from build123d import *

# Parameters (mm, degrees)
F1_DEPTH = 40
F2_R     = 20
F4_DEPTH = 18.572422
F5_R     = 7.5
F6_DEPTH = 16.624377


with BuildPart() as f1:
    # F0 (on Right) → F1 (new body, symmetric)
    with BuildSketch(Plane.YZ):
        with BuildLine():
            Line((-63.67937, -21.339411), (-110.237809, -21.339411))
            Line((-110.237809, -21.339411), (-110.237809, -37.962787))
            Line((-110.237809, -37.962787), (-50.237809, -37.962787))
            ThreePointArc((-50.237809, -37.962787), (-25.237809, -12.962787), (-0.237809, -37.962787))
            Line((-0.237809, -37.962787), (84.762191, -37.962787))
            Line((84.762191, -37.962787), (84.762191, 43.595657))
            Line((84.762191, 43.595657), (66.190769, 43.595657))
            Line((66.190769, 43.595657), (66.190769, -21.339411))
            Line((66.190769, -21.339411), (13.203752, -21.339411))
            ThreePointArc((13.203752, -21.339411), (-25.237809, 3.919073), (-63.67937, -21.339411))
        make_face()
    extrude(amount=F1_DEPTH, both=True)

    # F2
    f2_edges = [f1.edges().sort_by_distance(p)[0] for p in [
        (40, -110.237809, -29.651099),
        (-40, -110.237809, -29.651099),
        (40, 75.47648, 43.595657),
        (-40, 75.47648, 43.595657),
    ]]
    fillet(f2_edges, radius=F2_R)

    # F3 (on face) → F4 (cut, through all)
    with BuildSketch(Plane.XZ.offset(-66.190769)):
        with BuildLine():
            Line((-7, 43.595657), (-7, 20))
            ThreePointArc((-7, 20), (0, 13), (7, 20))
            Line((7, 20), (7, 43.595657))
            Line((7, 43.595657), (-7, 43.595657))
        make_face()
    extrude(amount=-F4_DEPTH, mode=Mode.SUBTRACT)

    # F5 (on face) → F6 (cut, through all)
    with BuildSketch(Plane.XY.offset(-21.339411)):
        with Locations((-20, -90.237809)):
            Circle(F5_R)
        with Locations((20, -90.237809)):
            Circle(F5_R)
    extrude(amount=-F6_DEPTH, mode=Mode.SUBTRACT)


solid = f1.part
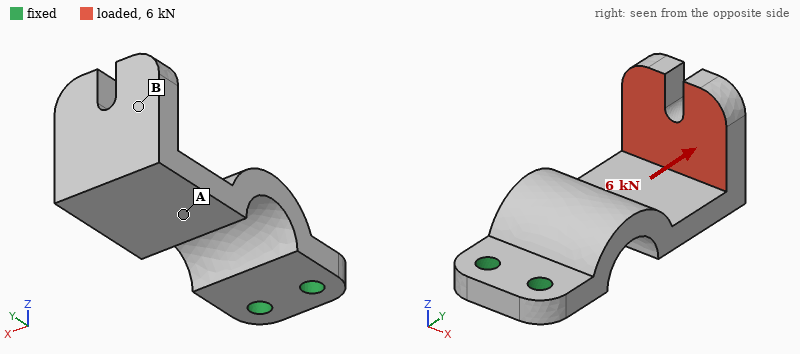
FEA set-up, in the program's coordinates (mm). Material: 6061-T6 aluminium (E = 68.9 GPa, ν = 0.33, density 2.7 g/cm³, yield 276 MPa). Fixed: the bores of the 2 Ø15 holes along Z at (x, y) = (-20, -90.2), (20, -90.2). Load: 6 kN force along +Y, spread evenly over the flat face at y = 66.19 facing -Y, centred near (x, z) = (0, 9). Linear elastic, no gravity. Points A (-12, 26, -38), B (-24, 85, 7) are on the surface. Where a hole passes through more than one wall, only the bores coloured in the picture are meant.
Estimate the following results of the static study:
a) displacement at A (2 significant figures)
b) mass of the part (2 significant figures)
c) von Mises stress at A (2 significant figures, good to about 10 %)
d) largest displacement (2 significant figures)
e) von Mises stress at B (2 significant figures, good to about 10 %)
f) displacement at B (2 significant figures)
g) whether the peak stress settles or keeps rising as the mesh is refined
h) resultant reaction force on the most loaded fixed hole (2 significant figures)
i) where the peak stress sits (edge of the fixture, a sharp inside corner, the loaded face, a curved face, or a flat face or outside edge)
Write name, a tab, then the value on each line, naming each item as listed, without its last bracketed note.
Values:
displacement at A	0.56 mm
mass of the part	1000 g
von Mises stress at A	51 MPa
largest displacement	1.7 mm
von Mises stress at B	11 MPa
displacement at B	1.4 mm
whether the peak stress settles or keeps rising as the mesh is refined	keeps rising
resultant reaction force on the most loaded fixed hole	3.1 kN
where the peak stress sits	edge of the fixture
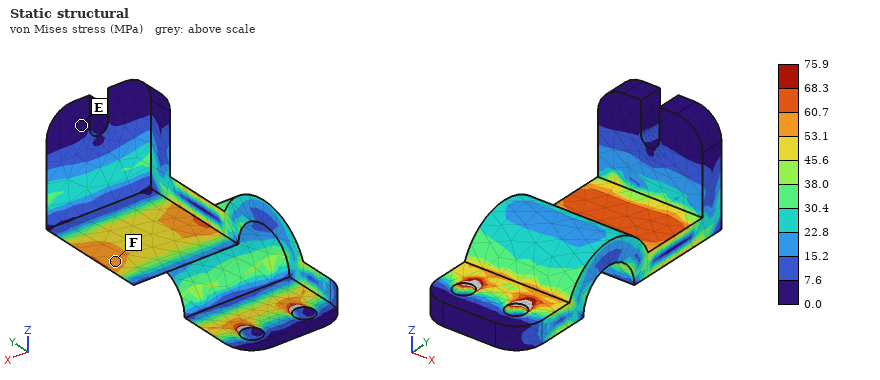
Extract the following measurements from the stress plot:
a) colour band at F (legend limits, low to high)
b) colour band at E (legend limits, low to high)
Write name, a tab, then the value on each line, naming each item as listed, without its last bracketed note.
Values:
colour band at F	53.1 to 60.7 MPa
colour band at E	0.0 to 7.6 MPa
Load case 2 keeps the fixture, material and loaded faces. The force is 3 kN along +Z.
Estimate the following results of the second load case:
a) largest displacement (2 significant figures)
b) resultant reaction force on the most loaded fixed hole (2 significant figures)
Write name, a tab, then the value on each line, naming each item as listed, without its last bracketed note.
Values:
largest displacement	2.4 mm
resultant reaction force on the most loaded fixed hole	1.6 kN
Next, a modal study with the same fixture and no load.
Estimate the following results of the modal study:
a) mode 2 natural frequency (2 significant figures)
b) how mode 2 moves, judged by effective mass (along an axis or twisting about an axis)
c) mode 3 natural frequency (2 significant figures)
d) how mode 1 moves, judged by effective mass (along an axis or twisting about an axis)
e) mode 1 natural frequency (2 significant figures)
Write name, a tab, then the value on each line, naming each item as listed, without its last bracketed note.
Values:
mode 2 natural frequency	760 Hz
how mode 2 moves, judged by effective mass	along X
mode 3 natural frequency	1100 Hz
how mode 1 moves, judged by effective mass	along Z
mode 1 natural frequency	280 Hz
